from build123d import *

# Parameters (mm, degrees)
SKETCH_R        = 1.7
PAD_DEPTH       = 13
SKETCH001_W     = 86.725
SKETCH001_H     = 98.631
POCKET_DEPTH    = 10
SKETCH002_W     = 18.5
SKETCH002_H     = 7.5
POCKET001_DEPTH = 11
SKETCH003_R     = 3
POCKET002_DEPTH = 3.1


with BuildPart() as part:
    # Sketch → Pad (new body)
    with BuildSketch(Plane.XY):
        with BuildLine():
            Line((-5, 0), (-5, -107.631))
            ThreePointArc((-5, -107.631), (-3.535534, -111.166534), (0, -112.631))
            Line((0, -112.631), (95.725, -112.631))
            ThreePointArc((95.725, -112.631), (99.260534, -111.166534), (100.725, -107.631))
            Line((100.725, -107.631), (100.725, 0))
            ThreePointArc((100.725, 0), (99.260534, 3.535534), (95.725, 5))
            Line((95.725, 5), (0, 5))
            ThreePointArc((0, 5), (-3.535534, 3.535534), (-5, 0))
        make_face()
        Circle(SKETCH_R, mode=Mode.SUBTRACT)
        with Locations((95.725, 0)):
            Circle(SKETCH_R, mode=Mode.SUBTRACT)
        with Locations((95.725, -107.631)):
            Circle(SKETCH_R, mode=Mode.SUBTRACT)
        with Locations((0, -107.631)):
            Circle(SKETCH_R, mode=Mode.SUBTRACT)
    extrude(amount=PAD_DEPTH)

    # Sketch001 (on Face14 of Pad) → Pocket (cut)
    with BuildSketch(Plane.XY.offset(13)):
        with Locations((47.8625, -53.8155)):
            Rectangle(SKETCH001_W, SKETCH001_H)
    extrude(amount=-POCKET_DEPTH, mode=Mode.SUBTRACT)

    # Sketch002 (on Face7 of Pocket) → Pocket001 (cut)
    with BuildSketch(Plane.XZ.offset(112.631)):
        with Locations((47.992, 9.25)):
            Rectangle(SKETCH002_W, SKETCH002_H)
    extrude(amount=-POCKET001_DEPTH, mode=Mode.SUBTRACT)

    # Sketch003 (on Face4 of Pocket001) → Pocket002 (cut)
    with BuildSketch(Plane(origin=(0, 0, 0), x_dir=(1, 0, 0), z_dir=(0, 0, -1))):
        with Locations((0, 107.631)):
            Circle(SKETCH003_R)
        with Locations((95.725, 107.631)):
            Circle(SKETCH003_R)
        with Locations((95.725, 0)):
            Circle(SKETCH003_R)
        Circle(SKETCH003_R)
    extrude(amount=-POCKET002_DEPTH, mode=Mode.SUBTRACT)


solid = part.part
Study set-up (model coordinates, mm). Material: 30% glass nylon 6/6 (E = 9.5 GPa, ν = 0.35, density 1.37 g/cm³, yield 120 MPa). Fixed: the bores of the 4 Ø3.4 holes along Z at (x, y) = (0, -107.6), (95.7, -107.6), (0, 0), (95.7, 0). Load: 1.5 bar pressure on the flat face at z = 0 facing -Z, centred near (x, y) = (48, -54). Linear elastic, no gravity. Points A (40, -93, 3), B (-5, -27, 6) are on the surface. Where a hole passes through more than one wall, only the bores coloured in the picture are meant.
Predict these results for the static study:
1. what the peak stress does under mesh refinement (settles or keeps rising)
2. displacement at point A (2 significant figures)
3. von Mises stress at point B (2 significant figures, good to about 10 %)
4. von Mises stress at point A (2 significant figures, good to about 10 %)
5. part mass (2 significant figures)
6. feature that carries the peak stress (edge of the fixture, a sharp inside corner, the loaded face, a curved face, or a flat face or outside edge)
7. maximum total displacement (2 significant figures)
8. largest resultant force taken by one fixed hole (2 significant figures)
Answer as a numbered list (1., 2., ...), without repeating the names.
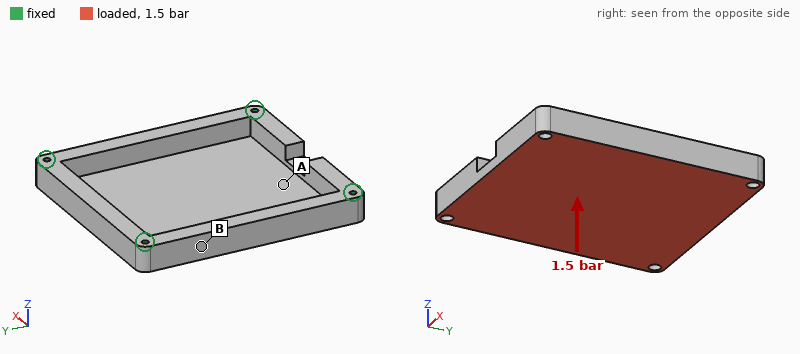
1. keeps rising
2. 0.35 mm
3. 6.1 MPa
4. 8.6 MPa
5. 100 g
6. edge of the fixture
7. 0.98 mm
8. 850 N
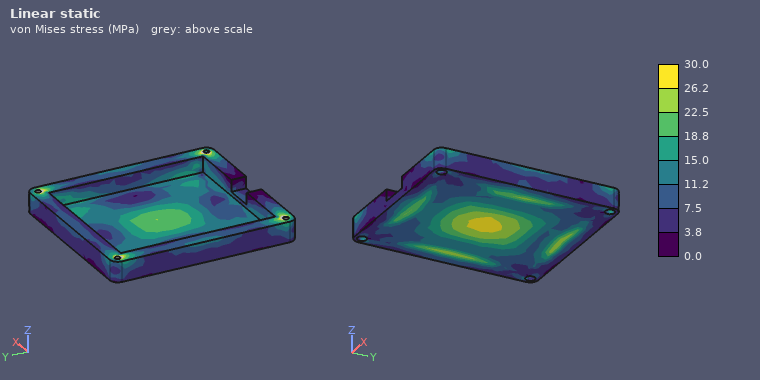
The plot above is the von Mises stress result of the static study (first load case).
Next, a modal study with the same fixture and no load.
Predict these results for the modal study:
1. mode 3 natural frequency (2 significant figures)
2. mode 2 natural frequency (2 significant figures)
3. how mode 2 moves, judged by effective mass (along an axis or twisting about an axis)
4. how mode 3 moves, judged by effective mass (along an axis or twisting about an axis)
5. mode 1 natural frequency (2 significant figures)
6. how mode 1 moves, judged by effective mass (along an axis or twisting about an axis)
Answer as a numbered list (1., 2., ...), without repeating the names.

1. 2200 Hz
2. 2100 Hz
3. twisting about Y
4. twisting about X
5. 1200 Hz
6. along Z
